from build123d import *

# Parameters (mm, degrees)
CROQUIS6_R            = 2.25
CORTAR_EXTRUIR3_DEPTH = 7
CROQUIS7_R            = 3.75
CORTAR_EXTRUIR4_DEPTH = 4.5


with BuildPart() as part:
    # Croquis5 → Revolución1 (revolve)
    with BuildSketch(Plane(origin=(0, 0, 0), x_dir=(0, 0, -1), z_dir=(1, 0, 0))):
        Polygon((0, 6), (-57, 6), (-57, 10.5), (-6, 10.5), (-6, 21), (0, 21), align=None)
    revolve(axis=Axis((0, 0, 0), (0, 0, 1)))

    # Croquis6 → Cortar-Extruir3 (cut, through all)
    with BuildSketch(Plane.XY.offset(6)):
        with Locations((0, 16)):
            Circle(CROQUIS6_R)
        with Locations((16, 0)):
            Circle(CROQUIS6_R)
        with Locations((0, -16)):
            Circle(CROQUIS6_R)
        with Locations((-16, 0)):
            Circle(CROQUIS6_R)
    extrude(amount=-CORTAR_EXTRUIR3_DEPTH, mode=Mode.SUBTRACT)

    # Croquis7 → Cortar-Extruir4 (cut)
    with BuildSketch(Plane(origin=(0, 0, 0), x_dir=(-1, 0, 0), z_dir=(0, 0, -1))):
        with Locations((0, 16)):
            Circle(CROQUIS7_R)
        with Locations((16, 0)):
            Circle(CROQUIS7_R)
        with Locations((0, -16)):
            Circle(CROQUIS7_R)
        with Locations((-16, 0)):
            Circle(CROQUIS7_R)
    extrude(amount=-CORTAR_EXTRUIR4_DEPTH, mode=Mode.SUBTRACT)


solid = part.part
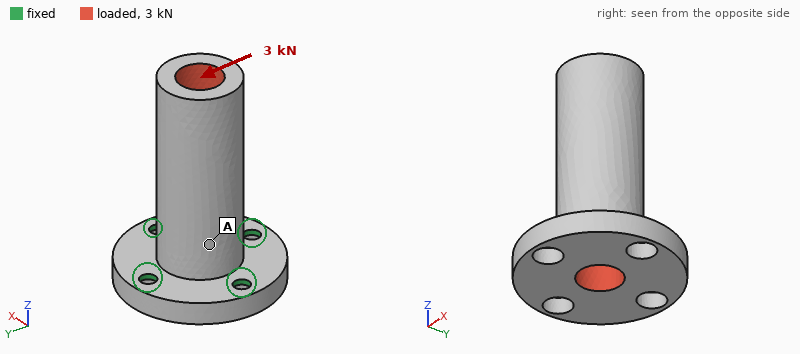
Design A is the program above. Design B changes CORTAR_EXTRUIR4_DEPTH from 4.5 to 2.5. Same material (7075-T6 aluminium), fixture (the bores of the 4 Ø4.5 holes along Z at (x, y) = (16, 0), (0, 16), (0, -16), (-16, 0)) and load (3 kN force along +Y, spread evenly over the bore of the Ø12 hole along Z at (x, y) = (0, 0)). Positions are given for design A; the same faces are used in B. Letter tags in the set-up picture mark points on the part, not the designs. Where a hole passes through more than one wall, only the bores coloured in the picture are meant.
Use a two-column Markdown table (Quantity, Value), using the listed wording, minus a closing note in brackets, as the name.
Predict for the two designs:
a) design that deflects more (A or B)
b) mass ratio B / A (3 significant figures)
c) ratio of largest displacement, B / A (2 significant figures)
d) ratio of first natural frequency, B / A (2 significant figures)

| Quantity | Value |
|---|---|
| design that deflects more | A |
| mass ratio B / A | 1.01 |
| ratio of largest displacement, B / A | 0.81 |
| ratio of first natural frequency, B / A | 1.1 |
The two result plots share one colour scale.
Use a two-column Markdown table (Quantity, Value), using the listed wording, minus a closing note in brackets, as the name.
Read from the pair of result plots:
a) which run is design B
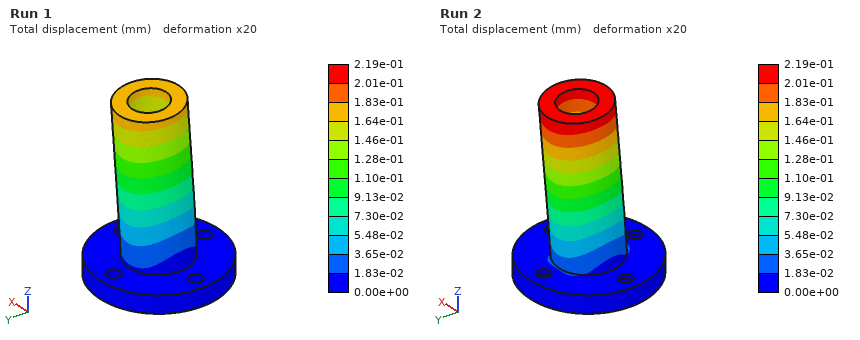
| Quantity | Value |
|---|---|
| which run is design B | Run 1 |
